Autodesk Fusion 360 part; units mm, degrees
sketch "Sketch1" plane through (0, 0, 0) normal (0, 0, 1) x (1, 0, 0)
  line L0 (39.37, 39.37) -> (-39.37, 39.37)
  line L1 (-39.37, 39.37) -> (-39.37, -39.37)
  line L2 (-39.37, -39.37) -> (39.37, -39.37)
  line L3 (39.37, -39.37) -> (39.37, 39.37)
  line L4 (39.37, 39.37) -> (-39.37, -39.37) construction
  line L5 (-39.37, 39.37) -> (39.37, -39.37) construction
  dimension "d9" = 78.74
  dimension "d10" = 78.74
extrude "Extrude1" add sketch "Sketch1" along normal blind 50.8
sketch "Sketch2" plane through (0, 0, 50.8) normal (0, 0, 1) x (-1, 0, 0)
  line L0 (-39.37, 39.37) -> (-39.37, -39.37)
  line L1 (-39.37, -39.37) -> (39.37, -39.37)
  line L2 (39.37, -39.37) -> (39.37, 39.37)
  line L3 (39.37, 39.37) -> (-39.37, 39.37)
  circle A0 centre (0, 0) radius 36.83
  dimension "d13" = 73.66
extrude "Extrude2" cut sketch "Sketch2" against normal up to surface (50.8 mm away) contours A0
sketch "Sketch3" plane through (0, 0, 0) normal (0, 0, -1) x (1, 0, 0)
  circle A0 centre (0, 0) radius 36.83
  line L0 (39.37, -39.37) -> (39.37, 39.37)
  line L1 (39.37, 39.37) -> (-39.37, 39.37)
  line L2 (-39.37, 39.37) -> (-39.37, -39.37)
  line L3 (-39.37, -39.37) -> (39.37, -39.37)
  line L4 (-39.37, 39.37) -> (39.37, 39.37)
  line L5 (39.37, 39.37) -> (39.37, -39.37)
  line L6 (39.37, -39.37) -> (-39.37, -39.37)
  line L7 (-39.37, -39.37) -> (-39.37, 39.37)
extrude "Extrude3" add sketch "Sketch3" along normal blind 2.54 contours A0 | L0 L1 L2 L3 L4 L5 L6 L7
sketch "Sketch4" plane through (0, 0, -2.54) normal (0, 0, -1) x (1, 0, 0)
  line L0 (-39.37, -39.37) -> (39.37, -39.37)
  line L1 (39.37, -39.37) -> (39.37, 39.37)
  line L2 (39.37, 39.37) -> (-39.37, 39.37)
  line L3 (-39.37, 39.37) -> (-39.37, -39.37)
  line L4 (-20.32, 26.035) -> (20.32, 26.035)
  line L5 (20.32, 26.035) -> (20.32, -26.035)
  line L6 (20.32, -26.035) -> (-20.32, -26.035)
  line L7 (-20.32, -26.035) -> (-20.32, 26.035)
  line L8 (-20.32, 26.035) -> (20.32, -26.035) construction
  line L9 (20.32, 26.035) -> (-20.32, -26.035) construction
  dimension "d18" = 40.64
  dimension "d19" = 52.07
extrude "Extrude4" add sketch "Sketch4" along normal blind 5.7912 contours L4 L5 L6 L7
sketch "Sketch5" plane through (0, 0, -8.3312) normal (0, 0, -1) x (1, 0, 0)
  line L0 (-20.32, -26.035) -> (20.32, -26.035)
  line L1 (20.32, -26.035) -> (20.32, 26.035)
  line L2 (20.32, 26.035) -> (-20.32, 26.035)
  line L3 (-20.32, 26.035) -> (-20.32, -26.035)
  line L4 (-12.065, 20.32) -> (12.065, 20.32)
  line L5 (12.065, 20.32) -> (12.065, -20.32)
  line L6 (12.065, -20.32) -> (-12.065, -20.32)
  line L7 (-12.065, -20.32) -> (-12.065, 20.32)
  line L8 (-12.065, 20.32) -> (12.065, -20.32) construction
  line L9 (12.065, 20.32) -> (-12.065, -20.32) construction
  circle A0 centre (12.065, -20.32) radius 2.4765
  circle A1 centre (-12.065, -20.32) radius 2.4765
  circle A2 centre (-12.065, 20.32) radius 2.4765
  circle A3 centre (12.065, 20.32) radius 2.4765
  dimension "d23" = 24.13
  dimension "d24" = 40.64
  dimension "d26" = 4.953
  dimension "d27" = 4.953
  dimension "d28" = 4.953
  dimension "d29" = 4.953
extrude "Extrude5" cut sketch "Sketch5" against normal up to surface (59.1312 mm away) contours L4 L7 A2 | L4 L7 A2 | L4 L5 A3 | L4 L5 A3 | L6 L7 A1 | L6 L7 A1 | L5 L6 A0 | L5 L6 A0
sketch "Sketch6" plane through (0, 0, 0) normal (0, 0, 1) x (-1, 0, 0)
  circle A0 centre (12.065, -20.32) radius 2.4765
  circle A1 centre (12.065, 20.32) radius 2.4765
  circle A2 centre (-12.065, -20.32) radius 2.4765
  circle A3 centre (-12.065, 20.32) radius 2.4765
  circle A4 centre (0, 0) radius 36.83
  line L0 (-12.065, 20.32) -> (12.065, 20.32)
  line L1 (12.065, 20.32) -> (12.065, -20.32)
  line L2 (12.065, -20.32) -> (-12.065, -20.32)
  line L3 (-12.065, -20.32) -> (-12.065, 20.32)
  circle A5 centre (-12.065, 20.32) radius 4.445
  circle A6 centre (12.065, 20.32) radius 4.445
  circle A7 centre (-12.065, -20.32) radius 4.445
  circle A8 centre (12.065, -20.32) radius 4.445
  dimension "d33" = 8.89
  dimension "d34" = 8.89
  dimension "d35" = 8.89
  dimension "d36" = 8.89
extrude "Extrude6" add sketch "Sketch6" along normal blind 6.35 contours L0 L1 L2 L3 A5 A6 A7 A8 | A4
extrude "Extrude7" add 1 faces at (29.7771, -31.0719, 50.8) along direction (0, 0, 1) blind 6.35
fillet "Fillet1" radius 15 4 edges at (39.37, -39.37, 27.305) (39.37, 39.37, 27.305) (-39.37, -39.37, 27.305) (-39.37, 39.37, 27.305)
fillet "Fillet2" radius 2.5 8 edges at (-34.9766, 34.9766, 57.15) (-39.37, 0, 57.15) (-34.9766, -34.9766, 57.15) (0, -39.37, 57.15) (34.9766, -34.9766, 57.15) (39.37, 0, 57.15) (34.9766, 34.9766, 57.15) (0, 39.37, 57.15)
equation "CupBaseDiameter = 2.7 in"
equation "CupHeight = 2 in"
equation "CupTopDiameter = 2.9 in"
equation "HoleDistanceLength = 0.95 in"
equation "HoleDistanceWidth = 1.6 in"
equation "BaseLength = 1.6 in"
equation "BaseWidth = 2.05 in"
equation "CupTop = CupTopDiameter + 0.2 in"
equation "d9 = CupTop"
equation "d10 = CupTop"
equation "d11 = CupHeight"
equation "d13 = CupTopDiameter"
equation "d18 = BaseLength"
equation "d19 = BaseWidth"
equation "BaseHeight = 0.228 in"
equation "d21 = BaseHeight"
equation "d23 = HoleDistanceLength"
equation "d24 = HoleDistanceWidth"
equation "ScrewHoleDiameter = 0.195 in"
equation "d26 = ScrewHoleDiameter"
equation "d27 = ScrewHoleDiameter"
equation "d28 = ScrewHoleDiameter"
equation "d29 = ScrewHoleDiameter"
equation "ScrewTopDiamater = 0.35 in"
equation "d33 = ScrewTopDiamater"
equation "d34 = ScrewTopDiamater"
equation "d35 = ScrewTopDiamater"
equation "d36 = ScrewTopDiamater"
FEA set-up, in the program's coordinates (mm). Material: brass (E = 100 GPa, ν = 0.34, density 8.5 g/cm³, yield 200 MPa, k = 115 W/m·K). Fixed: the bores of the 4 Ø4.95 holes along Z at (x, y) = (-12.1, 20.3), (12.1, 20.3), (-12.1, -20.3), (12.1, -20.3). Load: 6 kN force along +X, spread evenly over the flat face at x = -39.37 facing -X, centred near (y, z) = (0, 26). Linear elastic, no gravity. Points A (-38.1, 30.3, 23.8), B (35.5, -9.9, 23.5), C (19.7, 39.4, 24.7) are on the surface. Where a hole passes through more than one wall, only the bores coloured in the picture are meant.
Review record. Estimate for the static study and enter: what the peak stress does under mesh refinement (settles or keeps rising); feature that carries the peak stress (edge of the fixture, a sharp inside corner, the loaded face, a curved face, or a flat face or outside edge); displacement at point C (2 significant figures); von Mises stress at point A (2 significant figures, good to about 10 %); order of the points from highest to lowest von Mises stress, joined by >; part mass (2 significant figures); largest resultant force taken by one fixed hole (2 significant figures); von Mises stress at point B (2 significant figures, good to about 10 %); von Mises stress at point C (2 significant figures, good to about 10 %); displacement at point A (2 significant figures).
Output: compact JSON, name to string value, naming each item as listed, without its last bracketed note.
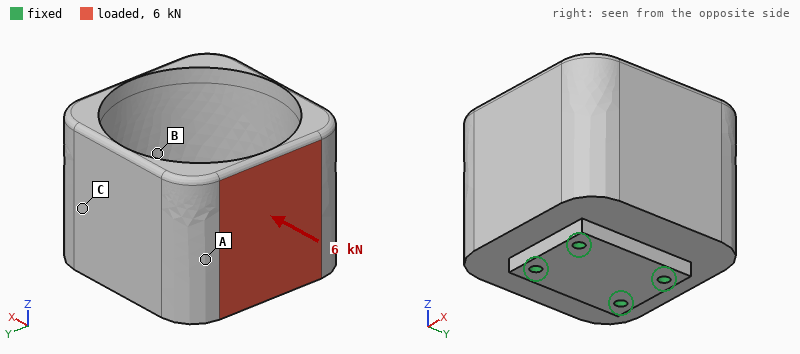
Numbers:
{"what the peak stress does under mesh refinement": "keeps rising", "feature that carries the peak stress": "edge of the fixture", "displacement at point C": "0.027 mm", "von Mises stress at point A": "32 MPa", "order of the points from highest to lowest von Mises stress, joined by >": "A > C > B", "part mass": "1.3 kg", "largest resultant force taken by one fixed hole": "3.4 kN", "von Mises stress at point B": "9.3 MPa", "von Mises stress at point C": "20 MPa", "displacement at point A": "0.039 mm"}
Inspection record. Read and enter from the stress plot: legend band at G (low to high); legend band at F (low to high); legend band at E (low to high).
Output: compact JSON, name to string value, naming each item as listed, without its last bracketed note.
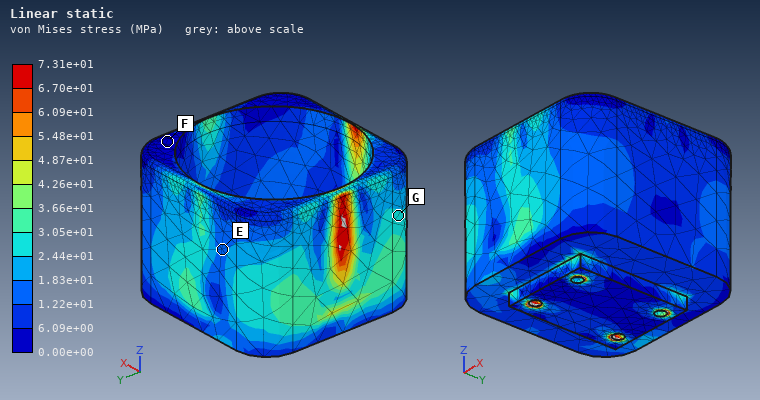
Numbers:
{"legend band at G": "2.44e+01 to 3.05e+01 MPa", "legend band at F": "0.00e+00 to 6.09e+00 MPa", "legend band at E": "1.22e+01 to 1.83e+01 MPa"}
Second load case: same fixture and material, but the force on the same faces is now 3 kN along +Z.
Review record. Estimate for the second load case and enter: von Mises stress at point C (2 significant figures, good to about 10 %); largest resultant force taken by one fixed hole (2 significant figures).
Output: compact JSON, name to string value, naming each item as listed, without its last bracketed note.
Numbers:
{"von Mises stress at point C": "5.7 MPa", "largest resultant force taken by one fixed hole": "2.8 kN"}
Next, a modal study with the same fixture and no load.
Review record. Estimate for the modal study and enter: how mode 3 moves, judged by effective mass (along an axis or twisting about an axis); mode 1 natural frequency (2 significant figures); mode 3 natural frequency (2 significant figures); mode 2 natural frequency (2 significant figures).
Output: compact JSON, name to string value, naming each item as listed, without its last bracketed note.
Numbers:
{"how mode 3 moves, judged by effective mass": "along Y", "mode 1 natural frequency": "1900 Hz", "mode 3 natural frequency": "2400 Hz", "mode 2 natural frequency": "1900 Hz"}
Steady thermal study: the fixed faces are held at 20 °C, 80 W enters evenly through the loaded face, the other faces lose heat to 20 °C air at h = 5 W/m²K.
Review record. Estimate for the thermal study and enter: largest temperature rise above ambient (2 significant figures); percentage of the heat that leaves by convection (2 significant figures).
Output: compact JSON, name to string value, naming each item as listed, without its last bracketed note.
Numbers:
{"largest temperature rise above ambient": "42 K", "percentage of the heat that leaves by convection": "3.2 %"}
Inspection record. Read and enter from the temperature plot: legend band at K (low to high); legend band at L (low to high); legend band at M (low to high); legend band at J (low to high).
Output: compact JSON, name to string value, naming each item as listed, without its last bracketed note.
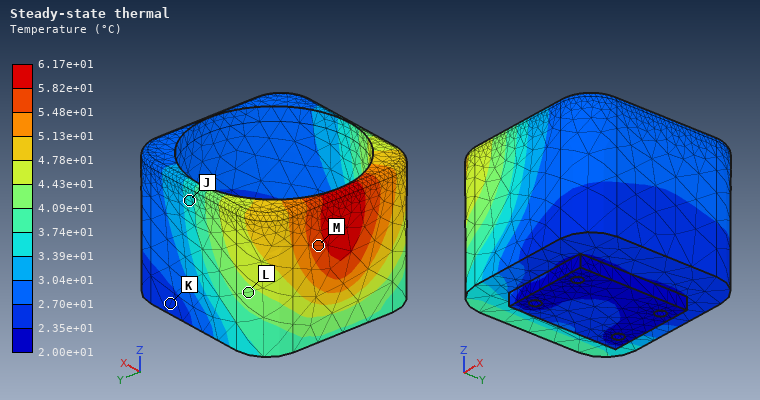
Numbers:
{"legend band at K": "2.35e+01 to 2.70e+01 °C", "legend band at L": "4.09e+01 to 4.43e+01 °C", "legend band at M": "5.48e+01 to 5.82e+01 °C", "legend band at J": "3.39e+01 to 3.74e+01 °C"}
